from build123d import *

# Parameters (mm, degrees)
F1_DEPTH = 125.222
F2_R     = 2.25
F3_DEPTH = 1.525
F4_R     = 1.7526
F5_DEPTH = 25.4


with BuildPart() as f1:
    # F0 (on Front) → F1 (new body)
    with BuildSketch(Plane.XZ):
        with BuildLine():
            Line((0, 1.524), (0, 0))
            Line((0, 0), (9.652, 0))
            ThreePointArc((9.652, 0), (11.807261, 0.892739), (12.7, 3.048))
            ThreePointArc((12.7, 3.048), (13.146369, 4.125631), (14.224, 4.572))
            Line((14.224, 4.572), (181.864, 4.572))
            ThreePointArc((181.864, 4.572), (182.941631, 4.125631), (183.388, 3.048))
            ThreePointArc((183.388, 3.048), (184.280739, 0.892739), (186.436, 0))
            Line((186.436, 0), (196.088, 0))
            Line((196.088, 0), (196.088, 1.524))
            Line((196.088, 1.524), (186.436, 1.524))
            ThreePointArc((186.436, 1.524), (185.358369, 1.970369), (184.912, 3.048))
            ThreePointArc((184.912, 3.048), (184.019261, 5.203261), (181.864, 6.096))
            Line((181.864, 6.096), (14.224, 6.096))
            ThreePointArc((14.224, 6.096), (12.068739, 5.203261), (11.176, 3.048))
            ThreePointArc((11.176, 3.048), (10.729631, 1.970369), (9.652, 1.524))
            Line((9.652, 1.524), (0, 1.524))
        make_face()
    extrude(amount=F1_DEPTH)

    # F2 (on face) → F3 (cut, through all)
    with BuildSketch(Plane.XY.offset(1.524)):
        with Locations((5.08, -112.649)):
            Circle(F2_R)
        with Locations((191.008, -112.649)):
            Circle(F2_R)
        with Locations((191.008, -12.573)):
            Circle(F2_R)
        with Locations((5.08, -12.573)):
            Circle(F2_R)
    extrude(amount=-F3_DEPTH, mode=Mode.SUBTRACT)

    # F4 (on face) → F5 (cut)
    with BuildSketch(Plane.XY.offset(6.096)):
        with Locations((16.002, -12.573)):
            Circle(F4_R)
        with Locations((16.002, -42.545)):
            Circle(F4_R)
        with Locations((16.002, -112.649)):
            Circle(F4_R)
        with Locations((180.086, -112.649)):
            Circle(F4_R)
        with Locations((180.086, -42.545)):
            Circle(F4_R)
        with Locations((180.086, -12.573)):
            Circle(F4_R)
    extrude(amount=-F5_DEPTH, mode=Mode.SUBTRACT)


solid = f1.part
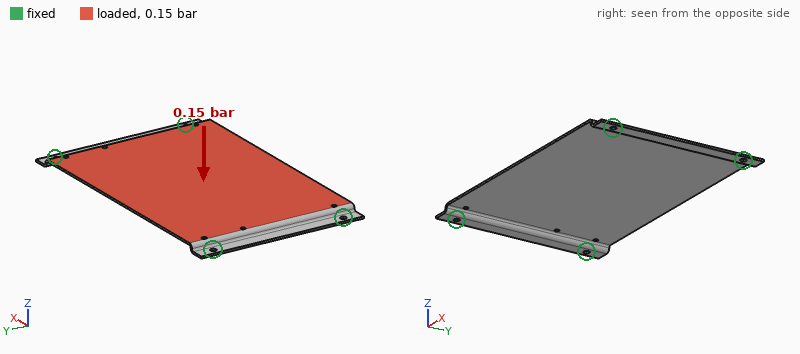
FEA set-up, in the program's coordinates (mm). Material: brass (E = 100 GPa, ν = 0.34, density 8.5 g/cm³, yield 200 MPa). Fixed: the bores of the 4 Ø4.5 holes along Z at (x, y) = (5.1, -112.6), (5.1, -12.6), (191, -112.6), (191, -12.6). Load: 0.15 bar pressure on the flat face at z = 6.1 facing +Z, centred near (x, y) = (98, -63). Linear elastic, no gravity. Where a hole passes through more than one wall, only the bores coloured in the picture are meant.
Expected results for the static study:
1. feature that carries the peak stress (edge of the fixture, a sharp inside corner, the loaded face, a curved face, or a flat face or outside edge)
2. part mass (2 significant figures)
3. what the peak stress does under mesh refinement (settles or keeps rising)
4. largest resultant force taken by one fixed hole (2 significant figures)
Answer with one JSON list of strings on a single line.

["a sharp inside corner", "320 g", "keeps rising", "570 N"]
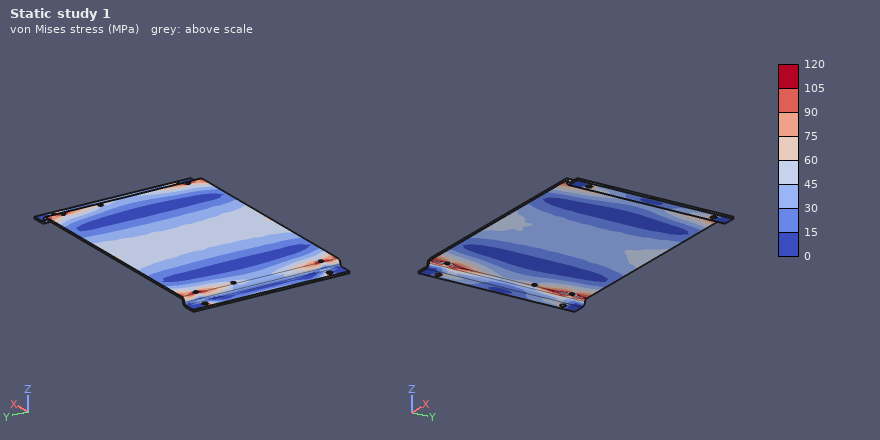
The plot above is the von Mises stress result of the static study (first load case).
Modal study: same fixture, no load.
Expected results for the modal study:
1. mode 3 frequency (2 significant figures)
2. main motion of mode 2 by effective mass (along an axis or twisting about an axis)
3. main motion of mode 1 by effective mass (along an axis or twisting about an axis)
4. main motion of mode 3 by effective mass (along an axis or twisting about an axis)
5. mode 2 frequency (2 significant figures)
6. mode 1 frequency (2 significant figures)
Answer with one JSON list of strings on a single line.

["390 Hz", "twisting about X", "along Z", "twisting about Y", "240 Hz", "170 Hz"]
